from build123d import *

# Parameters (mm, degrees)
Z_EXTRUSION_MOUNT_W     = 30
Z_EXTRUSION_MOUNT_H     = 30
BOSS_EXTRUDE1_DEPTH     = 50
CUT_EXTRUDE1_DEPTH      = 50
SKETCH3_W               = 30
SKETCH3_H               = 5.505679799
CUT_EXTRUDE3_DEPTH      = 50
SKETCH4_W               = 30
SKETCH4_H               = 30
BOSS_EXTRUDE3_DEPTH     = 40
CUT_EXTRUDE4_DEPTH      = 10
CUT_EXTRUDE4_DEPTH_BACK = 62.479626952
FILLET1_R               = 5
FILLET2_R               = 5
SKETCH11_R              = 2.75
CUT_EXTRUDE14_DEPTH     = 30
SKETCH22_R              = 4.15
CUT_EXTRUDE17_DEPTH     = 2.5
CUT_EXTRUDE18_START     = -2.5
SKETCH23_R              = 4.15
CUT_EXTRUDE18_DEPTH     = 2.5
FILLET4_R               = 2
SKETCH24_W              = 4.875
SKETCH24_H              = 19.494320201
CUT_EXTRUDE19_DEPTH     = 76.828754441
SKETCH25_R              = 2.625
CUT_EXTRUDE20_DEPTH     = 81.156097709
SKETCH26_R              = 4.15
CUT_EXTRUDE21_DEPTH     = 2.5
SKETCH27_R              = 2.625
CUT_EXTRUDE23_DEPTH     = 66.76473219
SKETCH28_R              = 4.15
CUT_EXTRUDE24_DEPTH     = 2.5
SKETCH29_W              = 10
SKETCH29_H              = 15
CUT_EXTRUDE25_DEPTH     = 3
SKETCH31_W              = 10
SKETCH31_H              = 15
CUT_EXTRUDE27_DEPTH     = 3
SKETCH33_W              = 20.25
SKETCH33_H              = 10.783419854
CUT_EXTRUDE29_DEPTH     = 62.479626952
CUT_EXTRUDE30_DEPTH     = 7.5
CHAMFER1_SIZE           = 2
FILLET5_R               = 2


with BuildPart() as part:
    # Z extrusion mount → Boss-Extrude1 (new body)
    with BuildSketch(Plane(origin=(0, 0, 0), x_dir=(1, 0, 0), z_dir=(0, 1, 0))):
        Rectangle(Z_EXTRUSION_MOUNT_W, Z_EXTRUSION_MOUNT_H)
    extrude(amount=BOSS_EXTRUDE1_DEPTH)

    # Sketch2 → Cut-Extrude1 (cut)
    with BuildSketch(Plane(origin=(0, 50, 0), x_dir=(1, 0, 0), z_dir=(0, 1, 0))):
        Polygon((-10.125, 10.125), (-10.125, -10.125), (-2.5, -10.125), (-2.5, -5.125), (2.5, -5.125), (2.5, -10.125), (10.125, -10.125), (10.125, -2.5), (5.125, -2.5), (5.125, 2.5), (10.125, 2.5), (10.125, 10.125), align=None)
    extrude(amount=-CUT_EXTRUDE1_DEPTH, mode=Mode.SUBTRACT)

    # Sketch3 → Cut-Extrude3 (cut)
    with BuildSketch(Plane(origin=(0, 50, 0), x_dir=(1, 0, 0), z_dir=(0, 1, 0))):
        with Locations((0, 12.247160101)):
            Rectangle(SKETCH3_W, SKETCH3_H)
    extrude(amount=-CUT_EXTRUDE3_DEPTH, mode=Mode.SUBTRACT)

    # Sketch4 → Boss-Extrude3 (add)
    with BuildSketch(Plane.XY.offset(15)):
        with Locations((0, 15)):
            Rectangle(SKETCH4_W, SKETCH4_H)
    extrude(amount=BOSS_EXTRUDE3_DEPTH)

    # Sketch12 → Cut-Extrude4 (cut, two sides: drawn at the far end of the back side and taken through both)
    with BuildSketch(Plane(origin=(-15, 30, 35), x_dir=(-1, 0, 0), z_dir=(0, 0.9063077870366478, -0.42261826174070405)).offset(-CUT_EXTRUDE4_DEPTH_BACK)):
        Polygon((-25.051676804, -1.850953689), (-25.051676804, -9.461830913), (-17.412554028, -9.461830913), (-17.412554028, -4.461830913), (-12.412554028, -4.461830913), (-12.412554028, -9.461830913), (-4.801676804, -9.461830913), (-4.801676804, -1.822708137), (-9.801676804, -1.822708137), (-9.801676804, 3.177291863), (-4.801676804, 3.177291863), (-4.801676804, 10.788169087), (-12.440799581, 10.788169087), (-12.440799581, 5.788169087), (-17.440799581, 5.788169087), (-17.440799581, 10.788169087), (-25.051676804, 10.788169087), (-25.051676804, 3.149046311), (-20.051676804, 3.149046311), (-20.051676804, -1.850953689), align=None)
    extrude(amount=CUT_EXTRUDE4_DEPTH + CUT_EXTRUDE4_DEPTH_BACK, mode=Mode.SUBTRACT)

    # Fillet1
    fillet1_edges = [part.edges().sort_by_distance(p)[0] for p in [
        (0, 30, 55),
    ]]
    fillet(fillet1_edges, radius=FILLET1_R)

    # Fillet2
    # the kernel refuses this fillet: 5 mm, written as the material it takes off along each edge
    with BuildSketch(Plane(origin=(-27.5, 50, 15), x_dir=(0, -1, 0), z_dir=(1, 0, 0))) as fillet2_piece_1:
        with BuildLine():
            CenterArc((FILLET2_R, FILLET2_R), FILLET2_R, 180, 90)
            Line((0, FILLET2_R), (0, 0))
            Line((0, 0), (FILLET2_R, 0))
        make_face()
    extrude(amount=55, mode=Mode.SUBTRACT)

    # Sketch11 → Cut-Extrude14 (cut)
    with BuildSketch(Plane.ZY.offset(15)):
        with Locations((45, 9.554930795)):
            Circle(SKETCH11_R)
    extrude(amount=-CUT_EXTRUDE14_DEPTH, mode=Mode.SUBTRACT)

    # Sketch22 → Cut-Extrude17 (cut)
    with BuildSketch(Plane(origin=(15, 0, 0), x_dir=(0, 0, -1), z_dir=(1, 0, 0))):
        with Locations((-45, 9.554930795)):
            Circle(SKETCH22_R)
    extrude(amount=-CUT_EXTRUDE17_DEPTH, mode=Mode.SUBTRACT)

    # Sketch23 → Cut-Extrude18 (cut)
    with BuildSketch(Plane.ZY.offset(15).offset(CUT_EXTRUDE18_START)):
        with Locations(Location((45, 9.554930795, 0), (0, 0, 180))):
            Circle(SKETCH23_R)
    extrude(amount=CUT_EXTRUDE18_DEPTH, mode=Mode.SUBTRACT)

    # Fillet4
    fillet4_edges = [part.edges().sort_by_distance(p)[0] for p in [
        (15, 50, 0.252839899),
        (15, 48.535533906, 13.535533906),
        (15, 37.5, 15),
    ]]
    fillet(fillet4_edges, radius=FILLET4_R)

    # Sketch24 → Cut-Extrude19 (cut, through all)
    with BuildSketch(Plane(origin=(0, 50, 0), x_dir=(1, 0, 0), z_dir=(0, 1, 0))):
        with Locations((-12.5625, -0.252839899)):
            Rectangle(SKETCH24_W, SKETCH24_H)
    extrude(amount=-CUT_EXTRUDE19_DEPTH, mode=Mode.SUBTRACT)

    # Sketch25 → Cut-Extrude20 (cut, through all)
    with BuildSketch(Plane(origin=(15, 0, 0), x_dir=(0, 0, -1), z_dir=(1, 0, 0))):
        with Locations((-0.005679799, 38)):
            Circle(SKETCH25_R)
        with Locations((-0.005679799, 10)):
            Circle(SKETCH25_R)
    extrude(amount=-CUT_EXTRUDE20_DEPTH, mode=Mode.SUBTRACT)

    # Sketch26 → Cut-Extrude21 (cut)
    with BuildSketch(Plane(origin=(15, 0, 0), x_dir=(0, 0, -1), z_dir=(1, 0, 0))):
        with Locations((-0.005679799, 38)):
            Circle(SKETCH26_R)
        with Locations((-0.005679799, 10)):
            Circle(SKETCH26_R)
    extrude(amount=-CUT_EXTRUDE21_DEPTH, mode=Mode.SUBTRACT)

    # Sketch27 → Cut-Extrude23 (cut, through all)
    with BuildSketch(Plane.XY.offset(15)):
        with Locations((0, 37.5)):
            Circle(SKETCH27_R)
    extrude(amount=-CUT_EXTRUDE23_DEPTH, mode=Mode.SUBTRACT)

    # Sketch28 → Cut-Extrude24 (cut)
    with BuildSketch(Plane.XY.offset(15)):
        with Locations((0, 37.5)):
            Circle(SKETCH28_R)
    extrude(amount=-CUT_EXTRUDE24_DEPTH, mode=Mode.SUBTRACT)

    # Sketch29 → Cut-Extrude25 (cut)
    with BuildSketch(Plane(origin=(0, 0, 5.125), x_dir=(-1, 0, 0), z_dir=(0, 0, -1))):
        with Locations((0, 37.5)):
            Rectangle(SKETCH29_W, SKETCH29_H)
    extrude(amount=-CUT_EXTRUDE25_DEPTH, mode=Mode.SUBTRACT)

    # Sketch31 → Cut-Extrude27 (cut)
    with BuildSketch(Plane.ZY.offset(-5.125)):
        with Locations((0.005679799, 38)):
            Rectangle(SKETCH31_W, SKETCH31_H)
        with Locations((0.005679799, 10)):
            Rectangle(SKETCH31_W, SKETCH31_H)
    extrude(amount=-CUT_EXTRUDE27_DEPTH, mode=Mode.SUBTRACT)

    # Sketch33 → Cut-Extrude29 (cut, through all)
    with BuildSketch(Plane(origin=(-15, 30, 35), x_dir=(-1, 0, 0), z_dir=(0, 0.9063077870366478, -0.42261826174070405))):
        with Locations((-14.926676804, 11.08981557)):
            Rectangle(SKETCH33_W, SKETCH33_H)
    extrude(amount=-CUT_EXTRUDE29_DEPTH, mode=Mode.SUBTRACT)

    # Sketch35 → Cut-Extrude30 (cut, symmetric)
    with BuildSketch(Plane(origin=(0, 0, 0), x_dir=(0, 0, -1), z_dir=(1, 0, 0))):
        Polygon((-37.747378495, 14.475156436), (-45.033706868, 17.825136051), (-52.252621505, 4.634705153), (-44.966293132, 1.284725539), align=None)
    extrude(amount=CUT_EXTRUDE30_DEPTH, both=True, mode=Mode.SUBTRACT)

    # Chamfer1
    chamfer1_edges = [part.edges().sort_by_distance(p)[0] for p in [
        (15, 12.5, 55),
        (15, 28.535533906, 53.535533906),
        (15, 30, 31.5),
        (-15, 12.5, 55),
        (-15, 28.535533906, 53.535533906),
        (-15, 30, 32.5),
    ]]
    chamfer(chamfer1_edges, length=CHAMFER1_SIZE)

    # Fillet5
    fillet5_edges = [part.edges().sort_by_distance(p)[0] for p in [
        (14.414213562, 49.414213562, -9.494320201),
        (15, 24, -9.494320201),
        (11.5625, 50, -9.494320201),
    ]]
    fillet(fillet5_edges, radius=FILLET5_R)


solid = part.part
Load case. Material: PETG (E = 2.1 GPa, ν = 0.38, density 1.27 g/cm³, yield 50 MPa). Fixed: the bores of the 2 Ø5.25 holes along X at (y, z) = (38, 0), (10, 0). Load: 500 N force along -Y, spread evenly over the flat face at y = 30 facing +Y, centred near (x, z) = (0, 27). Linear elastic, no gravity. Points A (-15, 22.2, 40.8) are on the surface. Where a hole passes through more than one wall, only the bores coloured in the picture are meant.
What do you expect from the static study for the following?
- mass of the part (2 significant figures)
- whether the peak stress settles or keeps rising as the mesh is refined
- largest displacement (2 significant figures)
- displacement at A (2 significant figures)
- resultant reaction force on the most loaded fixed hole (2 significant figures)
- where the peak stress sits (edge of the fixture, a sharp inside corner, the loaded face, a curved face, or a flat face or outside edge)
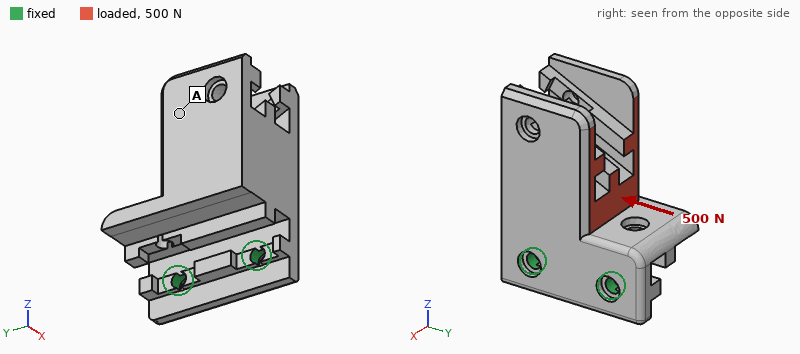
46 g
keeps rising
0.76 mm
0.60 mm
550 N
edge of the fixture
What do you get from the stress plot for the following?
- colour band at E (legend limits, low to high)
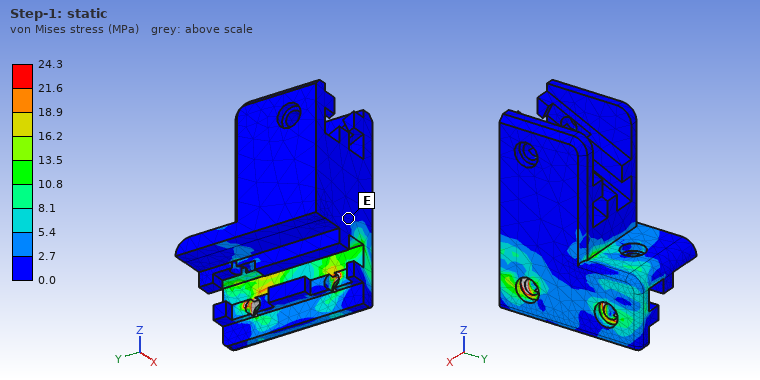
0.0 to 2.7 MPa
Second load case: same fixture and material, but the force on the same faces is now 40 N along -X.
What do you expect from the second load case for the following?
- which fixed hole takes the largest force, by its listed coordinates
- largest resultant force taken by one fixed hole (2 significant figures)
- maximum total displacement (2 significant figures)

(38, 0)
27 N
0.94 mm
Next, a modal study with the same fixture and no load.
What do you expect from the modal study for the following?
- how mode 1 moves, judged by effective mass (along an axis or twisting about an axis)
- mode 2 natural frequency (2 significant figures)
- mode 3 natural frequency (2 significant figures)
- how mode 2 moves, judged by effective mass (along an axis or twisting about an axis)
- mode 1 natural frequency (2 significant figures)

along X
840 Hz
1500 Hz
along Y
210 Hz
